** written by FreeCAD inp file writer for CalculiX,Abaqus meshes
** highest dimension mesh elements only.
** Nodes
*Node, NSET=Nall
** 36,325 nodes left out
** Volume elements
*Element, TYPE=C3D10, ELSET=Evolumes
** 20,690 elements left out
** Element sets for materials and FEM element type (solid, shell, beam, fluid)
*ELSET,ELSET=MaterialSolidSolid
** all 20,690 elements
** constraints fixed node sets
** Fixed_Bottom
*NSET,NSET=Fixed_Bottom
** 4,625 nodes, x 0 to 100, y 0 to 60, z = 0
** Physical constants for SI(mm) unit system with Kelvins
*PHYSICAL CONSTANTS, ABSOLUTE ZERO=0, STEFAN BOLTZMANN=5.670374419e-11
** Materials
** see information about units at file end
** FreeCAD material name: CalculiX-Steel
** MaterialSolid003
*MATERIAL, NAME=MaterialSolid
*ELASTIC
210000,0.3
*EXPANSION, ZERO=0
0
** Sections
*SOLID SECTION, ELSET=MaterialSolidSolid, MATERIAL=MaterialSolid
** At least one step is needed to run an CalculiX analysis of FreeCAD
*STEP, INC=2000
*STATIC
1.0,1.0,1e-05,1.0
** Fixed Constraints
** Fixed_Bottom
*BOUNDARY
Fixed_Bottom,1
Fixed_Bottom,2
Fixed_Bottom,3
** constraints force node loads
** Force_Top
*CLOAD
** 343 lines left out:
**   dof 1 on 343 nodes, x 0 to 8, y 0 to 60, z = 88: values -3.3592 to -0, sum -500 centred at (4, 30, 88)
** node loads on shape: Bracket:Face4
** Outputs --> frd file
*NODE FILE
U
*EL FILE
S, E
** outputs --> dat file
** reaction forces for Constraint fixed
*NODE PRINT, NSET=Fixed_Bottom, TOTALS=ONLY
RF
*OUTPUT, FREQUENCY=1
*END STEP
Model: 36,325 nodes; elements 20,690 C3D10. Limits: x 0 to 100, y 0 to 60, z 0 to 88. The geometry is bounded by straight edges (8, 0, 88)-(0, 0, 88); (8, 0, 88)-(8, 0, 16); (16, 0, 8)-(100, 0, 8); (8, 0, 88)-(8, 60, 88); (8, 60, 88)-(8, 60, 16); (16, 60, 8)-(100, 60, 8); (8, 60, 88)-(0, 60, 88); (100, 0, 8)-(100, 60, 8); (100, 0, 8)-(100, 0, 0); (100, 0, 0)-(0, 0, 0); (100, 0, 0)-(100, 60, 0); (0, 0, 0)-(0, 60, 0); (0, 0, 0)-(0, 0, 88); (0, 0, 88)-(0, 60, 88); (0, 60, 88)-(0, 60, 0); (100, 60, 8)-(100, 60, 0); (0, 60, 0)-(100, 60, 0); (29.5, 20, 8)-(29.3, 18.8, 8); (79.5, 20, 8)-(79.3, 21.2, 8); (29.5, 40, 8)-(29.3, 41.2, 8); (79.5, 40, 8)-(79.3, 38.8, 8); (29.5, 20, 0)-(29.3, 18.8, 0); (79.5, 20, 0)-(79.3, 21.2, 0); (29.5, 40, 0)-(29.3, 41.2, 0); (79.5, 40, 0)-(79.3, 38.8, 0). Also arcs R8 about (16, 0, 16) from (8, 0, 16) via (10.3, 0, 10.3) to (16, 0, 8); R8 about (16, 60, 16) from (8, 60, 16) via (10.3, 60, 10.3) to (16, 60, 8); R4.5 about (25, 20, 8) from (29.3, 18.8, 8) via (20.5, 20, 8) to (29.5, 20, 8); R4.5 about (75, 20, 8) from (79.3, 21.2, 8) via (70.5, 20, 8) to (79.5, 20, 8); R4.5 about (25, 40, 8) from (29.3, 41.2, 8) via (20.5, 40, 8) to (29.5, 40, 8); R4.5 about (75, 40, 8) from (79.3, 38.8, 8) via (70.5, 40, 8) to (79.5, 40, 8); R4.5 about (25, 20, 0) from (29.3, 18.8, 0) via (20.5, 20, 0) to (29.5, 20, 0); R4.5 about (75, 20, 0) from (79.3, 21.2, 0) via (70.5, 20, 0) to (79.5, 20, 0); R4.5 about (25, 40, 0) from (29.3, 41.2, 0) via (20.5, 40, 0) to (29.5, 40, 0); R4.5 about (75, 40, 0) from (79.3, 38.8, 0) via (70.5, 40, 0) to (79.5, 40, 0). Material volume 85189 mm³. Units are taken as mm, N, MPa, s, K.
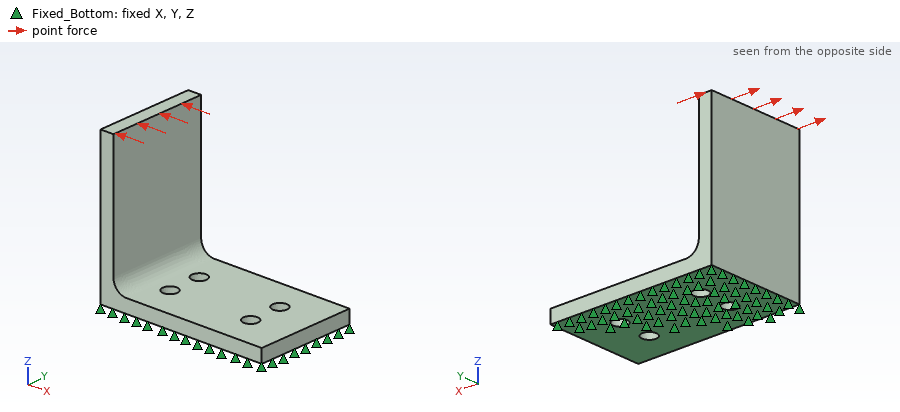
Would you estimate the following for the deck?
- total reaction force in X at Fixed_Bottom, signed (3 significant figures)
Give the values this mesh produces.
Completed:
500 N
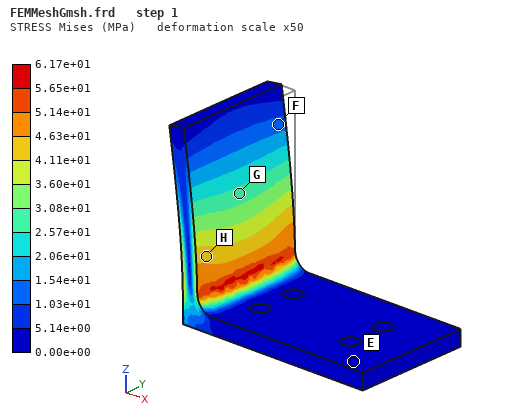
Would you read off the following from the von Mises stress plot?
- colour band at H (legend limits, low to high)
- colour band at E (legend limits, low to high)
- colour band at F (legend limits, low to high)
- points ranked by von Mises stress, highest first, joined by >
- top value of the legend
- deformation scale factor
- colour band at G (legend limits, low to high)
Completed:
4.11e+01 to 4.63e+01 MPa
0.00e+00 to 5.14e+00 MPa
1.03e+01 to 1.54e+01 MPa
H > G > F > E
6.17e+01 MPa
50
2.57e+01 to 3.08e+01 MPa
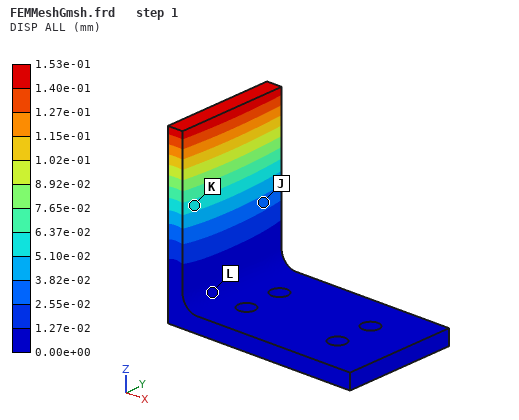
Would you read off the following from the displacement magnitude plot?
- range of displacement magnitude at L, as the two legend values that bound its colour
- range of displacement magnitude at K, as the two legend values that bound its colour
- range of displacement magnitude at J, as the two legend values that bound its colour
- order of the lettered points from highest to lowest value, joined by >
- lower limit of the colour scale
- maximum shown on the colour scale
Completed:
0.00e+00 to 1.27e-02 mm
5.10e-02 to 6.37e-02 mm
2.55e-02 to 3.82e-02 mm
K > J > L
0.00e+00 mm
1.53e-01 mm
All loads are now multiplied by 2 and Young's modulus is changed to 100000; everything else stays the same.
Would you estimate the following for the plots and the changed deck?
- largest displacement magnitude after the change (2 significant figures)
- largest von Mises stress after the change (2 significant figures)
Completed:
0.64 mm
120 MPa
